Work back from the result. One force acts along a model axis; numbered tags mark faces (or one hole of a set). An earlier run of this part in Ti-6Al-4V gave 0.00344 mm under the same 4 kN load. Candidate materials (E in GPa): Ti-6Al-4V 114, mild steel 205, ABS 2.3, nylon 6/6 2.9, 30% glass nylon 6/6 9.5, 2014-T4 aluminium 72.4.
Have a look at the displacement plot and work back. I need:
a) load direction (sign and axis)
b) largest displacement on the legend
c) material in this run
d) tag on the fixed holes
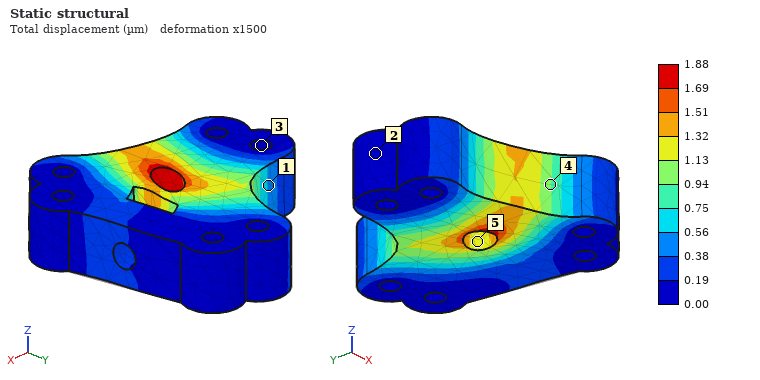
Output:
-Y
1.88 µm
mild steel
3
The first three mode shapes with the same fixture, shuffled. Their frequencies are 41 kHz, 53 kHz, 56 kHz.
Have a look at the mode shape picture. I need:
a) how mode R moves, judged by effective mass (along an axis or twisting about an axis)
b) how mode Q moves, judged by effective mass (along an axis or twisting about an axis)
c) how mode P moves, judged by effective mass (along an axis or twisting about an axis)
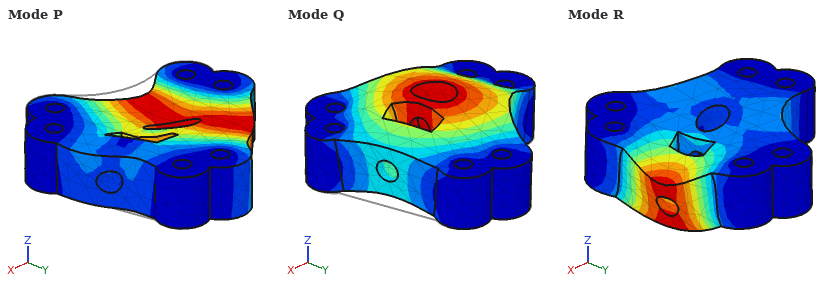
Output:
twisting about Y
along Z
along Y
